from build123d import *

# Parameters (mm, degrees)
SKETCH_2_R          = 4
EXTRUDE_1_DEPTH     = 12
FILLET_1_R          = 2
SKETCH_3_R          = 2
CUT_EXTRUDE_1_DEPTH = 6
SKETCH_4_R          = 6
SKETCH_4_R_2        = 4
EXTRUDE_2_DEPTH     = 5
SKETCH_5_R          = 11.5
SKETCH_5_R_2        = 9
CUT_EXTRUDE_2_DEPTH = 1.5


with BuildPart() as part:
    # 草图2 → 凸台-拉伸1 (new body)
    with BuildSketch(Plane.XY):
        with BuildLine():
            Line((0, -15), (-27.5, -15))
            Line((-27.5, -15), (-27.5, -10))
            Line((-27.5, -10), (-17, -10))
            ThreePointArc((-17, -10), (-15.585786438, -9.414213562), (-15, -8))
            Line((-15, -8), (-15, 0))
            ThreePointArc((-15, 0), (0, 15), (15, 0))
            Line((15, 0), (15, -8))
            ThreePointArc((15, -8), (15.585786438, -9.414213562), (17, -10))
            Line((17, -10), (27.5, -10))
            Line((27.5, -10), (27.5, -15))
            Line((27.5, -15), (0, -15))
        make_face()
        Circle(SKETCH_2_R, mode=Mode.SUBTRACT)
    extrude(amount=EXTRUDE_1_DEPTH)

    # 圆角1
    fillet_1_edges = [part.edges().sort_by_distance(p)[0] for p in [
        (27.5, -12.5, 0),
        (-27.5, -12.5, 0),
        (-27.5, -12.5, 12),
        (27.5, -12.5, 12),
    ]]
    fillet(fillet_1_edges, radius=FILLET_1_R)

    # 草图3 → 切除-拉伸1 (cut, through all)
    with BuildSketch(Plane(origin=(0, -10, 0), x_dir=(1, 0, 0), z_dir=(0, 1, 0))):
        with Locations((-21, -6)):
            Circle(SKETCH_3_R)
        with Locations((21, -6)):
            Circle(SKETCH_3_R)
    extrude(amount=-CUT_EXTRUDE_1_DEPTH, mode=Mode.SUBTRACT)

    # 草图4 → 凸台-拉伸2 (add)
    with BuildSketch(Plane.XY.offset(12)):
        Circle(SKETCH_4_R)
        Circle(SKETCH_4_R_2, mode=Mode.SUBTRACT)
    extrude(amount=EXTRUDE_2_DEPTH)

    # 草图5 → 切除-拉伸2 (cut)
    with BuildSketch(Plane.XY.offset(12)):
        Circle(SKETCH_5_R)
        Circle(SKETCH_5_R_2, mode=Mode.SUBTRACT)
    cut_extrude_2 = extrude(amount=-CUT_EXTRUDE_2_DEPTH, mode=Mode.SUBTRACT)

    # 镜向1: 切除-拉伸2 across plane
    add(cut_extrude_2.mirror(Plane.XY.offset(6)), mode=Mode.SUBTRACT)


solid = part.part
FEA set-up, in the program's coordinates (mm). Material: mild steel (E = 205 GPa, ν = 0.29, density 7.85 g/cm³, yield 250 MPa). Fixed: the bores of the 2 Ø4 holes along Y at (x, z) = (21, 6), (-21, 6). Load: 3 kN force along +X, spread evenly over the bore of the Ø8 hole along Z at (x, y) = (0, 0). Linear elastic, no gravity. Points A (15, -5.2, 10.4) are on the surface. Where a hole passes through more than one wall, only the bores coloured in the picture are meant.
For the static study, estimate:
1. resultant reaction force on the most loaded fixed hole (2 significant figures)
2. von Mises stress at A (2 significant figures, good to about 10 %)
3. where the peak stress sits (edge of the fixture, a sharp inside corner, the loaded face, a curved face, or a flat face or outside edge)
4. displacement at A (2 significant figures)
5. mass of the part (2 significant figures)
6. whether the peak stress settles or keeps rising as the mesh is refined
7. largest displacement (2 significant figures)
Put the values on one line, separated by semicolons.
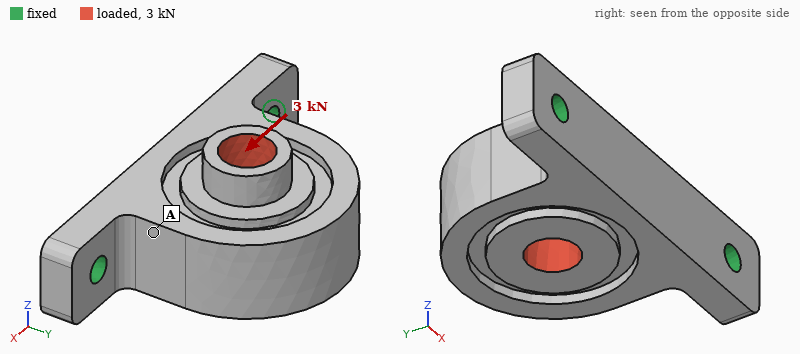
1.8 kN; 18 MPa; edge of the fixture; 3.7 µm; 80 g; keeps rising; 8.0 µm
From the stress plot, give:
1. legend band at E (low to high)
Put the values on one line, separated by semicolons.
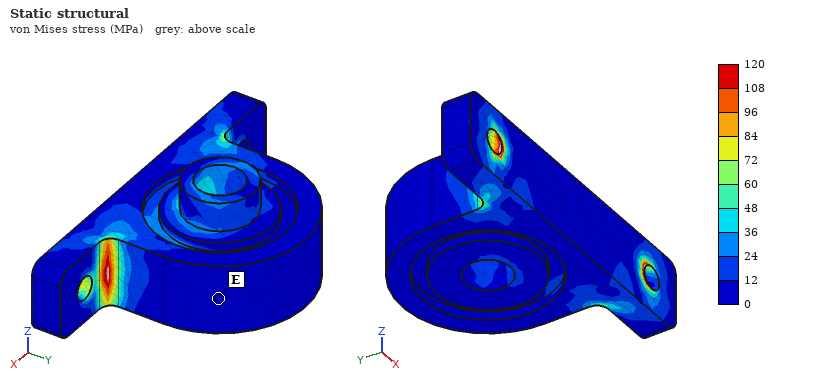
0 to 12 MPa
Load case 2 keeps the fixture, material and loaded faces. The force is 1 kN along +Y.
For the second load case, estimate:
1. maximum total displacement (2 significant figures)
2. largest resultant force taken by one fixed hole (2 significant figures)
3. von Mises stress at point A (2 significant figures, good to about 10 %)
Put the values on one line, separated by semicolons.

8.0 µm; 570 N; 14 MPa
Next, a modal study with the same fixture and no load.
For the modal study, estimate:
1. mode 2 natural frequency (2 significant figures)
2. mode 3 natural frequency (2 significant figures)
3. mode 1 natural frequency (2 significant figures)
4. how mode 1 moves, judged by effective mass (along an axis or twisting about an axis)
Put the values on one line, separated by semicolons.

14 kHz; 15 kHz; 4200 Hz; along Z
